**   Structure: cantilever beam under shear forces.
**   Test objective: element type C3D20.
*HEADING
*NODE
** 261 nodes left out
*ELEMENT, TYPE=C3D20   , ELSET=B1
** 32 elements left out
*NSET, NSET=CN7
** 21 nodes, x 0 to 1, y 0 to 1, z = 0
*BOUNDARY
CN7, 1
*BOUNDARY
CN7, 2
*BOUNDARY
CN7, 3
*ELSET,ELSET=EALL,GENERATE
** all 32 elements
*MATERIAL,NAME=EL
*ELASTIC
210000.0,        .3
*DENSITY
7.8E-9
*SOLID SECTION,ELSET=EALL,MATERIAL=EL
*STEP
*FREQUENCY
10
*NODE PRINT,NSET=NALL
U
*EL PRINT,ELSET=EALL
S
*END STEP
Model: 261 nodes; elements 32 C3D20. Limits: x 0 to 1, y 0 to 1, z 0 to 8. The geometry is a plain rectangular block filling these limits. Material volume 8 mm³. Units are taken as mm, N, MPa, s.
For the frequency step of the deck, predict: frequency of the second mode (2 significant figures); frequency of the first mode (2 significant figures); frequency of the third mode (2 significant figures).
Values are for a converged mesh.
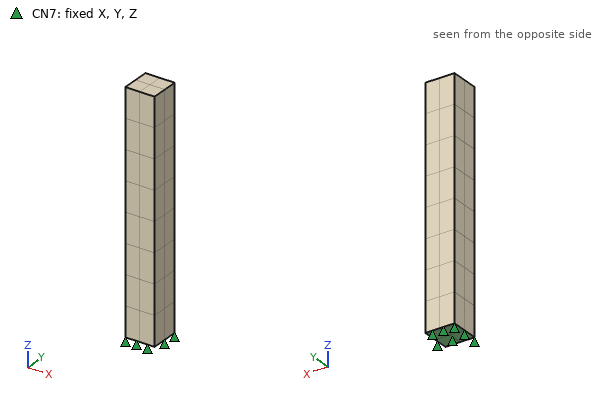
13000 Hz
13000 Hz
76000 Hz
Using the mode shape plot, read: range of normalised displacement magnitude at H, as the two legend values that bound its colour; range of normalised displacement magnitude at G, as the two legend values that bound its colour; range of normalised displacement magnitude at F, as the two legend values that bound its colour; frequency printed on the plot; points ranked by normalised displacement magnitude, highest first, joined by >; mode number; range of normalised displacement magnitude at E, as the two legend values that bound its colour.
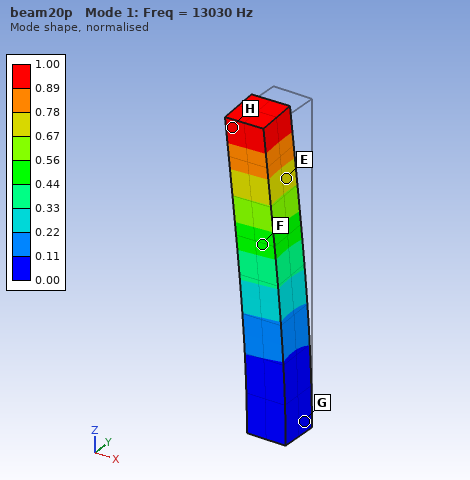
0.89 to 1.00
0.00 to 0.11
0.44 to 0.56
13030 Hz
H > E > F > G
1
0.67 to 0.78
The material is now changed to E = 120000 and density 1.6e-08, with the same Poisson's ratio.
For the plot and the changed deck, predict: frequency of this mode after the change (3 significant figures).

6870 Hz
